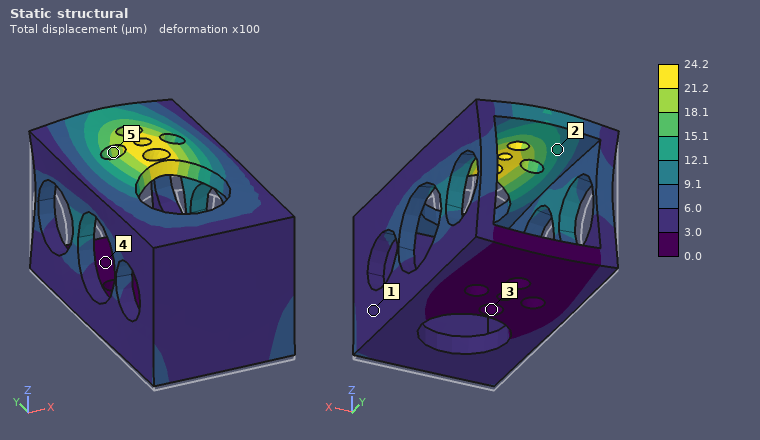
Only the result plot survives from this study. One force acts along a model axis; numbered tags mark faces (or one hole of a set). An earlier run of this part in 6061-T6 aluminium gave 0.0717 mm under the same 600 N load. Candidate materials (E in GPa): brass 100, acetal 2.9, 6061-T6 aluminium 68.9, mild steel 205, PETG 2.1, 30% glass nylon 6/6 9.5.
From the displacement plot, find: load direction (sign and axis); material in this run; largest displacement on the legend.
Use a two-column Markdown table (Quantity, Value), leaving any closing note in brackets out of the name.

| Quantity | Value |
|---|---|
| load direction | +Z |
| material in this run | mild steel |
| largest displacement on the legend | 24.2 µm |
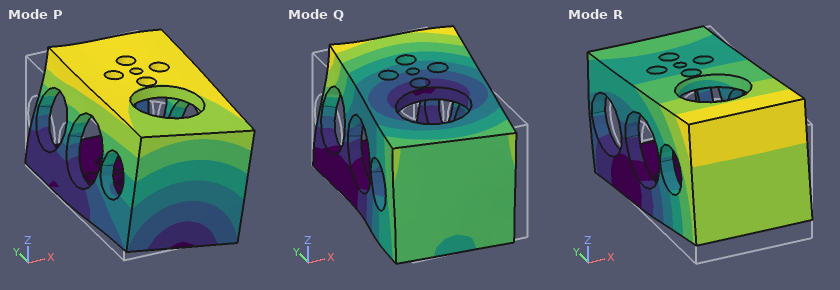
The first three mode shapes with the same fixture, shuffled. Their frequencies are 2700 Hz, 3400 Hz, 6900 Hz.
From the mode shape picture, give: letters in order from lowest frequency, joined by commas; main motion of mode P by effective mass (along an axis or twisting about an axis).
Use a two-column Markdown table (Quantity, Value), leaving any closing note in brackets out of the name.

| Quantity | Value |
|---|---|
| letters in order from lowest frequency, joined by commas | R, P, Q |
| main motion of mode P by effective mass | along X |
